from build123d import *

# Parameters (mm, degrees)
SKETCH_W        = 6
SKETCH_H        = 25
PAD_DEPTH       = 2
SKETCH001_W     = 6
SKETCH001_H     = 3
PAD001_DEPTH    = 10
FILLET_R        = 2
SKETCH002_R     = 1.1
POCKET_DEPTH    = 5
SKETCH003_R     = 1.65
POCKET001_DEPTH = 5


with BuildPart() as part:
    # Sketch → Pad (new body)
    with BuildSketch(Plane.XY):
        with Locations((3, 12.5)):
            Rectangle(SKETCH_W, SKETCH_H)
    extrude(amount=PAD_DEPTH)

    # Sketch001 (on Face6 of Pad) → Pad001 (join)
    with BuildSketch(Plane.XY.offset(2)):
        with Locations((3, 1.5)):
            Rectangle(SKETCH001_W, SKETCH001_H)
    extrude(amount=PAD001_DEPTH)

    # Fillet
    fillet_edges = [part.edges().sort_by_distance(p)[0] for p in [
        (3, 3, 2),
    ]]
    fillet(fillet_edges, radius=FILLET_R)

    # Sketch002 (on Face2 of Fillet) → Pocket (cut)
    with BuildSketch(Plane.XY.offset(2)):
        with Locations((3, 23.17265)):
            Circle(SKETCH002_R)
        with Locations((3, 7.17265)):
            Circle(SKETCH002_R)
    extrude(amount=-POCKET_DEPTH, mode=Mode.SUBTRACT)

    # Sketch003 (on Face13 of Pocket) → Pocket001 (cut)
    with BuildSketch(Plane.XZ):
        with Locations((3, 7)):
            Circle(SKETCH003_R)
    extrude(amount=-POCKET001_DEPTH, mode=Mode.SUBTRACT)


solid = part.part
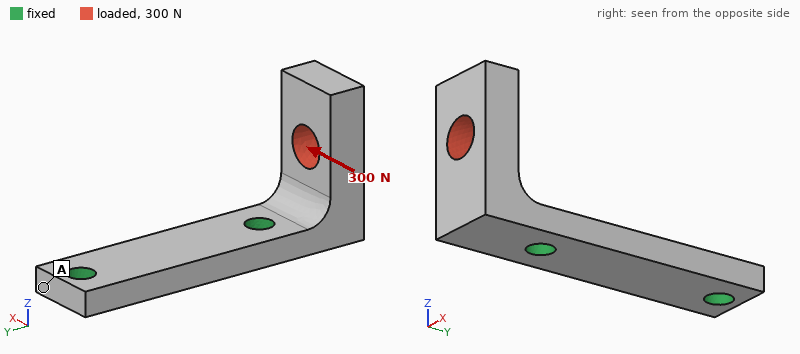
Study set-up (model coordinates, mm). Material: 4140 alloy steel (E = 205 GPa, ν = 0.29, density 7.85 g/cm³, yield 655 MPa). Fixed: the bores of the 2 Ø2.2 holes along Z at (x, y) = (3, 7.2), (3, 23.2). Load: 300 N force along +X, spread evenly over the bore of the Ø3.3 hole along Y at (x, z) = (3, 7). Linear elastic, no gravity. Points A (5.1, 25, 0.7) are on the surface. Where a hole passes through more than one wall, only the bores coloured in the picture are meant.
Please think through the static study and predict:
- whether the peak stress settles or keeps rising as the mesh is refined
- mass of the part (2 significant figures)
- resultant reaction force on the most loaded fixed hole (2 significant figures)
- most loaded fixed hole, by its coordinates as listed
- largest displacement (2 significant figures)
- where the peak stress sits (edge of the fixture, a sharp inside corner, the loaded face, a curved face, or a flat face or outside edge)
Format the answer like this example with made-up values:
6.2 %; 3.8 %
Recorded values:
keeps rising; 3.5 g; 340 N; (3, 7.2); 62 µm; edge of the fixture
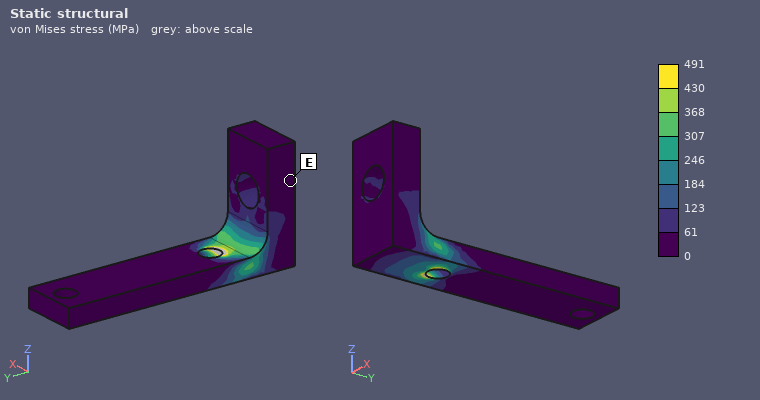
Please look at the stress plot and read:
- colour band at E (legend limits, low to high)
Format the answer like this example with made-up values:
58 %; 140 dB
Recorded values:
0 to 61 MPa
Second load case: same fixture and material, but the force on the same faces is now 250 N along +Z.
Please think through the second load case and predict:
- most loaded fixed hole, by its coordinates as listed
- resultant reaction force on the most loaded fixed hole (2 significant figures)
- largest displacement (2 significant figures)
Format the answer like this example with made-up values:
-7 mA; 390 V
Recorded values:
(3, 7.2); 250 N; 44 µm
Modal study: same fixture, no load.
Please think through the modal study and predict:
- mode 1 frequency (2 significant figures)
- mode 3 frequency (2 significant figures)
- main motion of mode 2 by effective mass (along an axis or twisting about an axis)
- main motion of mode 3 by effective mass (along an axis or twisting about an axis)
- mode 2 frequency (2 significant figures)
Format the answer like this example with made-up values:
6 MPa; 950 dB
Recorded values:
8500 Hz; 32 kHz; along X; along Z; 12 kHz
